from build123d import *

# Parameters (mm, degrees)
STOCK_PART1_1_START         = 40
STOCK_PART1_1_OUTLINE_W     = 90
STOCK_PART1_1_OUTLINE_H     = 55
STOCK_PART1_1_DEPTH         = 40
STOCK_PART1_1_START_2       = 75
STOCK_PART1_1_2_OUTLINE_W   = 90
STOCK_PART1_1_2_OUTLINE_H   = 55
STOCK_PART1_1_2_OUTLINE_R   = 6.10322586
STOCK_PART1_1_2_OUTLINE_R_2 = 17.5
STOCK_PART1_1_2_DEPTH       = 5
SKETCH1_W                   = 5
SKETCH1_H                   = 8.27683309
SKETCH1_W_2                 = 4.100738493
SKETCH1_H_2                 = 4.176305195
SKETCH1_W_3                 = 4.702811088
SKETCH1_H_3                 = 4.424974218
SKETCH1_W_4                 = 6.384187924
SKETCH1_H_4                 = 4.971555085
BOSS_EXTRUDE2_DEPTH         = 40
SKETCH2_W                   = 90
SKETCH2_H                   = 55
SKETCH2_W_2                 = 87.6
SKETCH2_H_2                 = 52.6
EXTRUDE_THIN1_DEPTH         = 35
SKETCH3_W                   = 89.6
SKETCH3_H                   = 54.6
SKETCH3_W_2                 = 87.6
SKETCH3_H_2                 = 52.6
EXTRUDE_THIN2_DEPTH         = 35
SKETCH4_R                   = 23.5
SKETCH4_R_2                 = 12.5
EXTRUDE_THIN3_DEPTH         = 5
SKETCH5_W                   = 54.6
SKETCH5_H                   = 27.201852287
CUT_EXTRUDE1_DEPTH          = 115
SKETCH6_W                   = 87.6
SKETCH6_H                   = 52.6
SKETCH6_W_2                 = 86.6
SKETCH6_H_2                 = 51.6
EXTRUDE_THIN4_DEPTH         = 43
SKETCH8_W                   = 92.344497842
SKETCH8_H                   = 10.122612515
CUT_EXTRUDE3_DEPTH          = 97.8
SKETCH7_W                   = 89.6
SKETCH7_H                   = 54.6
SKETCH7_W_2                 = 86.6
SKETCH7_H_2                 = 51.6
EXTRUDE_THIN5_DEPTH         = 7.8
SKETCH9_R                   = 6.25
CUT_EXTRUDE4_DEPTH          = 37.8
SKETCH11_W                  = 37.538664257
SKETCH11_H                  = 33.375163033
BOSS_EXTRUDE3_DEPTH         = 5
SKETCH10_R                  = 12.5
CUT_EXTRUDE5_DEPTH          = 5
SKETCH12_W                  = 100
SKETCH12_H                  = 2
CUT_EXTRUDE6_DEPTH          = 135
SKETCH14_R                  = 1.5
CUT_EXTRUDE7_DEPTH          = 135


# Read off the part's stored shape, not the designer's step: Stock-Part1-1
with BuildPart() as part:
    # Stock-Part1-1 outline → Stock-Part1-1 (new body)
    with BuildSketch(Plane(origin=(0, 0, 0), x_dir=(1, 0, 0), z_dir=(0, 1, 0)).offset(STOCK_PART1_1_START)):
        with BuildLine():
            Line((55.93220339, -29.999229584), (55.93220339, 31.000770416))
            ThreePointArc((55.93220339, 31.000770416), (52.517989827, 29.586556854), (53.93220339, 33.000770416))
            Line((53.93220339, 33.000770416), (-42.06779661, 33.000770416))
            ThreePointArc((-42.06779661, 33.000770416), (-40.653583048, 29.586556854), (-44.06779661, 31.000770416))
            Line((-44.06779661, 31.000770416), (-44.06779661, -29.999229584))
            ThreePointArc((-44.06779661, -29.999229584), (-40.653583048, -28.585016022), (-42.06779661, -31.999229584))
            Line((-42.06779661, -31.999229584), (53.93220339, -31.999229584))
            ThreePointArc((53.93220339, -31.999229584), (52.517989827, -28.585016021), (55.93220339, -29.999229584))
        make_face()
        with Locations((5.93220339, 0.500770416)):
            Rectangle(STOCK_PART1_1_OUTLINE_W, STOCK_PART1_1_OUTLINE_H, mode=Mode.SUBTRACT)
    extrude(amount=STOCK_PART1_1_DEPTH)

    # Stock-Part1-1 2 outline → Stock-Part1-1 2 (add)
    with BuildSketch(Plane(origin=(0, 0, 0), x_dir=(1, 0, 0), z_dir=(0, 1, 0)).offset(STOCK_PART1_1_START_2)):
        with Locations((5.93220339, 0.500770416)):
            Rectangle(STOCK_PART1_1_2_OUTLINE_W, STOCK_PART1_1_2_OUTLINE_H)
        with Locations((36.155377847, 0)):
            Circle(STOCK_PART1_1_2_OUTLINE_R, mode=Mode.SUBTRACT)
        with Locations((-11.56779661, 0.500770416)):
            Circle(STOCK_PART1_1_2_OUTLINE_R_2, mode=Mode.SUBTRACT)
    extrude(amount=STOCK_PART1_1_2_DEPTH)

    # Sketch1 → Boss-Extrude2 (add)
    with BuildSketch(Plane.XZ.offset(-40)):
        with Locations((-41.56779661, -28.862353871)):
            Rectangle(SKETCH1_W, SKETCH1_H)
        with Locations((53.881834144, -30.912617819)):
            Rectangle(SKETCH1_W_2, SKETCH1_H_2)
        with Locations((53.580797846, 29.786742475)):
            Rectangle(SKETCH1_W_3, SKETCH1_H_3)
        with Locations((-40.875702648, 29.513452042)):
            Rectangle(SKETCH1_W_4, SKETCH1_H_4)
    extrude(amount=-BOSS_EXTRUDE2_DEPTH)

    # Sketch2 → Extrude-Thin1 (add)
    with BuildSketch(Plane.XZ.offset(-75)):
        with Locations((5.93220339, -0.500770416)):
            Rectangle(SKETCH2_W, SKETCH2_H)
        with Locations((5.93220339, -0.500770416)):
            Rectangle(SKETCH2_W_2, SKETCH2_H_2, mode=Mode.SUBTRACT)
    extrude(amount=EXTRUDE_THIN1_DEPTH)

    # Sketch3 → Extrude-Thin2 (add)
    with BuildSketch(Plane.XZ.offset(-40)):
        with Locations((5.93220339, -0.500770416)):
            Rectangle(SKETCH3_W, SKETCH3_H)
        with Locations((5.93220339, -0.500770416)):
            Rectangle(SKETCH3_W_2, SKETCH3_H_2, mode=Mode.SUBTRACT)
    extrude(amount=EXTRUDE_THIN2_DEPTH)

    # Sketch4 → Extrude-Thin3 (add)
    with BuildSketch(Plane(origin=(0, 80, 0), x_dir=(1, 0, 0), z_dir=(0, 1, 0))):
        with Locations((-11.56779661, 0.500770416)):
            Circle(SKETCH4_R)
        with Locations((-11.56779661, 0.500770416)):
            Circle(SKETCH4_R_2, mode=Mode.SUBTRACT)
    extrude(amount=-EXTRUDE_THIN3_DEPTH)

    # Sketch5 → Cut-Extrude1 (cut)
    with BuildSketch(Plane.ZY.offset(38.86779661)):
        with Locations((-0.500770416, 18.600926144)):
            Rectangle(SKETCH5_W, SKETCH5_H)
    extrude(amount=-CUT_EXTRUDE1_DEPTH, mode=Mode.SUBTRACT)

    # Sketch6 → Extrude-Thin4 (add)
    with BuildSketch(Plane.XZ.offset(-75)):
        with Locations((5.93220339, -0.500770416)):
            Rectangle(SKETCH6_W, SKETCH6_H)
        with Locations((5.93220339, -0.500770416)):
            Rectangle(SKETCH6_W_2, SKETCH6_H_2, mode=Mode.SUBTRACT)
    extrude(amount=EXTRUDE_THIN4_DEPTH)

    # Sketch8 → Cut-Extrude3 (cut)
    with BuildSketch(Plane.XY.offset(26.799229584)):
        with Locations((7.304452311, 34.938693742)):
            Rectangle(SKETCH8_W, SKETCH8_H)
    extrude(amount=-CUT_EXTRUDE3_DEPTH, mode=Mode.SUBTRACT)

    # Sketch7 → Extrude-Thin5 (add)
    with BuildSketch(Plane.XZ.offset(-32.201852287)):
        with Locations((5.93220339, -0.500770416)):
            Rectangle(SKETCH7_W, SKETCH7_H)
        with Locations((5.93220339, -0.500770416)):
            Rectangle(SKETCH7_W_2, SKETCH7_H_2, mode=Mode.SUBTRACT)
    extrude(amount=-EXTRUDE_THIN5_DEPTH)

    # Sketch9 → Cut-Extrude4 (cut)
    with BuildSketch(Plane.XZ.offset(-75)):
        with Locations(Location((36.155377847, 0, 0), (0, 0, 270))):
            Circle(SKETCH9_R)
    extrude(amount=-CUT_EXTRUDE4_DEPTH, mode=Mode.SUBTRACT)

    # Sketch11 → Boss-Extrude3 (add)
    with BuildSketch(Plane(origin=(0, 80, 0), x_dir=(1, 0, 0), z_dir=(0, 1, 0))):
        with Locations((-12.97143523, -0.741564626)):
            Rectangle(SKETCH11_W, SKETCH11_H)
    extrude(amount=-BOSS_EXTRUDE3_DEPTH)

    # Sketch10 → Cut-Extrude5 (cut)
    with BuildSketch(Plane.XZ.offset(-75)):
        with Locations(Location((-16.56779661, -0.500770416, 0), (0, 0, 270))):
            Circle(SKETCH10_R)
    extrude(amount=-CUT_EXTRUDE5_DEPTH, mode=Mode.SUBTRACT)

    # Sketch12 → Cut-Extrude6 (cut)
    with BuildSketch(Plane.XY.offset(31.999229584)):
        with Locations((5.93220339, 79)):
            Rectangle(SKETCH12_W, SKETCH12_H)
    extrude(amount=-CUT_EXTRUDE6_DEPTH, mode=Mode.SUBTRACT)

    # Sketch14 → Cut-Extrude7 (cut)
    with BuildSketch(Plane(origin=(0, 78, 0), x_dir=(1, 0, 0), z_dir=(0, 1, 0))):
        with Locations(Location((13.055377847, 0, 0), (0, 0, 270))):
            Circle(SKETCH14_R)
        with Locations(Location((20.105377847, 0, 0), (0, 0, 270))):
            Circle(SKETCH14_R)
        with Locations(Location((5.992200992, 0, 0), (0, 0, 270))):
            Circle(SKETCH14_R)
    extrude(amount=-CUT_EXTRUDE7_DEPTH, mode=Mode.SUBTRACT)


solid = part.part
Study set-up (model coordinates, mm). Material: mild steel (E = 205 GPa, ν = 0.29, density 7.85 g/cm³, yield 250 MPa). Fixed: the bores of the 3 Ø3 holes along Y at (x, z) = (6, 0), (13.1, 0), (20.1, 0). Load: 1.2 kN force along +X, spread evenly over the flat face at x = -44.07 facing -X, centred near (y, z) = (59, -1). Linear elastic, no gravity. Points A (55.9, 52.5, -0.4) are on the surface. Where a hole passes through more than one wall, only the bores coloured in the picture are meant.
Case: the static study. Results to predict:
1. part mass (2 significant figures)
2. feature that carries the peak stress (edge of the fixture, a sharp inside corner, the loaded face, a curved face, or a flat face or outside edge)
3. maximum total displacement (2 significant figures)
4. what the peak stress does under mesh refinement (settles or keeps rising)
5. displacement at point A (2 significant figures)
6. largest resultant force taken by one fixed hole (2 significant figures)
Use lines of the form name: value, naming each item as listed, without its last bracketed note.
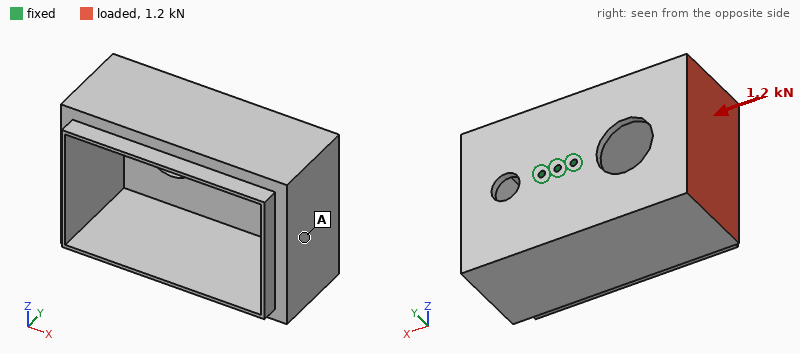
part mass: 720 g
feature that carries the peak stress: edge of the fixture
maximum total displacement: 0.24 mm
what the peak stress does under mesh refinement: keeps rising
displacement at point A: 0.16 mm
largest resultant force taken by one fixed hole: 1.1 kN
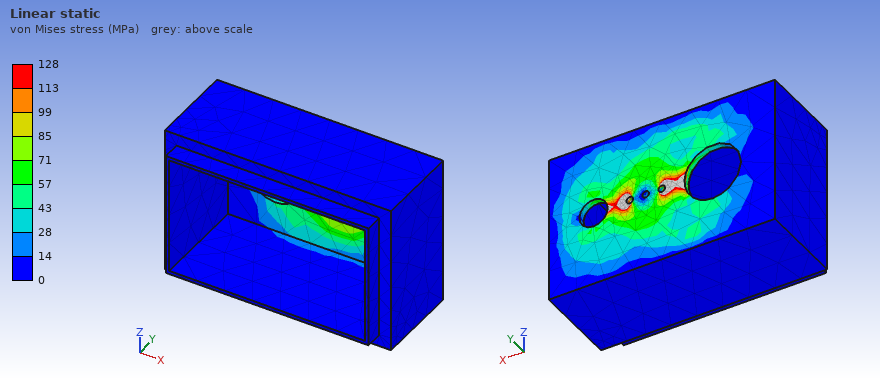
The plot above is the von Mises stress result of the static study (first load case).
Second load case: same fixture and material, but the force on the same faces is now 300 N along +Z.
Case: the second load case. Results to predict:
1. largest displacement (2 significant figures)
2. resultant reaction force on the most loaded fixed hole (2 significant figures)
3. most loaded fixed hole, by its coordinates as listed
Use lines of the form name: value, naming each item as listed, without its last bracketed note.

largest displacement: 77 µm
resultant reaction force on the most loaded fixed hole: 1.2 kN
most loaded fixed hole, by its coordinates as listed: (6, 0)
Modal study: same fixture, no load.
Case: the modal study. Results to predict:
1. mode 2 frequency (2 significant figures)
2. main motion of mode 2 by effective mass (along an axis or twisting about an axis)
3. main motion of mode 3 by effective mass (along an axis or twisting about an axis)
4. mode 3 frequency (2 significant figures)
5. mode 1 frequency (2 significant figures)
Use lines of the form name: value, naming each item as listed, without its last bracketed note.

mode 2 frequency: 390 Hz
main motion of mode 2 by effective mass: along Z
main motion of mode 3 by effective mass: along Y
mode 3 frequency: 1000 Hz
mode 1 frequency: 360 Hz
